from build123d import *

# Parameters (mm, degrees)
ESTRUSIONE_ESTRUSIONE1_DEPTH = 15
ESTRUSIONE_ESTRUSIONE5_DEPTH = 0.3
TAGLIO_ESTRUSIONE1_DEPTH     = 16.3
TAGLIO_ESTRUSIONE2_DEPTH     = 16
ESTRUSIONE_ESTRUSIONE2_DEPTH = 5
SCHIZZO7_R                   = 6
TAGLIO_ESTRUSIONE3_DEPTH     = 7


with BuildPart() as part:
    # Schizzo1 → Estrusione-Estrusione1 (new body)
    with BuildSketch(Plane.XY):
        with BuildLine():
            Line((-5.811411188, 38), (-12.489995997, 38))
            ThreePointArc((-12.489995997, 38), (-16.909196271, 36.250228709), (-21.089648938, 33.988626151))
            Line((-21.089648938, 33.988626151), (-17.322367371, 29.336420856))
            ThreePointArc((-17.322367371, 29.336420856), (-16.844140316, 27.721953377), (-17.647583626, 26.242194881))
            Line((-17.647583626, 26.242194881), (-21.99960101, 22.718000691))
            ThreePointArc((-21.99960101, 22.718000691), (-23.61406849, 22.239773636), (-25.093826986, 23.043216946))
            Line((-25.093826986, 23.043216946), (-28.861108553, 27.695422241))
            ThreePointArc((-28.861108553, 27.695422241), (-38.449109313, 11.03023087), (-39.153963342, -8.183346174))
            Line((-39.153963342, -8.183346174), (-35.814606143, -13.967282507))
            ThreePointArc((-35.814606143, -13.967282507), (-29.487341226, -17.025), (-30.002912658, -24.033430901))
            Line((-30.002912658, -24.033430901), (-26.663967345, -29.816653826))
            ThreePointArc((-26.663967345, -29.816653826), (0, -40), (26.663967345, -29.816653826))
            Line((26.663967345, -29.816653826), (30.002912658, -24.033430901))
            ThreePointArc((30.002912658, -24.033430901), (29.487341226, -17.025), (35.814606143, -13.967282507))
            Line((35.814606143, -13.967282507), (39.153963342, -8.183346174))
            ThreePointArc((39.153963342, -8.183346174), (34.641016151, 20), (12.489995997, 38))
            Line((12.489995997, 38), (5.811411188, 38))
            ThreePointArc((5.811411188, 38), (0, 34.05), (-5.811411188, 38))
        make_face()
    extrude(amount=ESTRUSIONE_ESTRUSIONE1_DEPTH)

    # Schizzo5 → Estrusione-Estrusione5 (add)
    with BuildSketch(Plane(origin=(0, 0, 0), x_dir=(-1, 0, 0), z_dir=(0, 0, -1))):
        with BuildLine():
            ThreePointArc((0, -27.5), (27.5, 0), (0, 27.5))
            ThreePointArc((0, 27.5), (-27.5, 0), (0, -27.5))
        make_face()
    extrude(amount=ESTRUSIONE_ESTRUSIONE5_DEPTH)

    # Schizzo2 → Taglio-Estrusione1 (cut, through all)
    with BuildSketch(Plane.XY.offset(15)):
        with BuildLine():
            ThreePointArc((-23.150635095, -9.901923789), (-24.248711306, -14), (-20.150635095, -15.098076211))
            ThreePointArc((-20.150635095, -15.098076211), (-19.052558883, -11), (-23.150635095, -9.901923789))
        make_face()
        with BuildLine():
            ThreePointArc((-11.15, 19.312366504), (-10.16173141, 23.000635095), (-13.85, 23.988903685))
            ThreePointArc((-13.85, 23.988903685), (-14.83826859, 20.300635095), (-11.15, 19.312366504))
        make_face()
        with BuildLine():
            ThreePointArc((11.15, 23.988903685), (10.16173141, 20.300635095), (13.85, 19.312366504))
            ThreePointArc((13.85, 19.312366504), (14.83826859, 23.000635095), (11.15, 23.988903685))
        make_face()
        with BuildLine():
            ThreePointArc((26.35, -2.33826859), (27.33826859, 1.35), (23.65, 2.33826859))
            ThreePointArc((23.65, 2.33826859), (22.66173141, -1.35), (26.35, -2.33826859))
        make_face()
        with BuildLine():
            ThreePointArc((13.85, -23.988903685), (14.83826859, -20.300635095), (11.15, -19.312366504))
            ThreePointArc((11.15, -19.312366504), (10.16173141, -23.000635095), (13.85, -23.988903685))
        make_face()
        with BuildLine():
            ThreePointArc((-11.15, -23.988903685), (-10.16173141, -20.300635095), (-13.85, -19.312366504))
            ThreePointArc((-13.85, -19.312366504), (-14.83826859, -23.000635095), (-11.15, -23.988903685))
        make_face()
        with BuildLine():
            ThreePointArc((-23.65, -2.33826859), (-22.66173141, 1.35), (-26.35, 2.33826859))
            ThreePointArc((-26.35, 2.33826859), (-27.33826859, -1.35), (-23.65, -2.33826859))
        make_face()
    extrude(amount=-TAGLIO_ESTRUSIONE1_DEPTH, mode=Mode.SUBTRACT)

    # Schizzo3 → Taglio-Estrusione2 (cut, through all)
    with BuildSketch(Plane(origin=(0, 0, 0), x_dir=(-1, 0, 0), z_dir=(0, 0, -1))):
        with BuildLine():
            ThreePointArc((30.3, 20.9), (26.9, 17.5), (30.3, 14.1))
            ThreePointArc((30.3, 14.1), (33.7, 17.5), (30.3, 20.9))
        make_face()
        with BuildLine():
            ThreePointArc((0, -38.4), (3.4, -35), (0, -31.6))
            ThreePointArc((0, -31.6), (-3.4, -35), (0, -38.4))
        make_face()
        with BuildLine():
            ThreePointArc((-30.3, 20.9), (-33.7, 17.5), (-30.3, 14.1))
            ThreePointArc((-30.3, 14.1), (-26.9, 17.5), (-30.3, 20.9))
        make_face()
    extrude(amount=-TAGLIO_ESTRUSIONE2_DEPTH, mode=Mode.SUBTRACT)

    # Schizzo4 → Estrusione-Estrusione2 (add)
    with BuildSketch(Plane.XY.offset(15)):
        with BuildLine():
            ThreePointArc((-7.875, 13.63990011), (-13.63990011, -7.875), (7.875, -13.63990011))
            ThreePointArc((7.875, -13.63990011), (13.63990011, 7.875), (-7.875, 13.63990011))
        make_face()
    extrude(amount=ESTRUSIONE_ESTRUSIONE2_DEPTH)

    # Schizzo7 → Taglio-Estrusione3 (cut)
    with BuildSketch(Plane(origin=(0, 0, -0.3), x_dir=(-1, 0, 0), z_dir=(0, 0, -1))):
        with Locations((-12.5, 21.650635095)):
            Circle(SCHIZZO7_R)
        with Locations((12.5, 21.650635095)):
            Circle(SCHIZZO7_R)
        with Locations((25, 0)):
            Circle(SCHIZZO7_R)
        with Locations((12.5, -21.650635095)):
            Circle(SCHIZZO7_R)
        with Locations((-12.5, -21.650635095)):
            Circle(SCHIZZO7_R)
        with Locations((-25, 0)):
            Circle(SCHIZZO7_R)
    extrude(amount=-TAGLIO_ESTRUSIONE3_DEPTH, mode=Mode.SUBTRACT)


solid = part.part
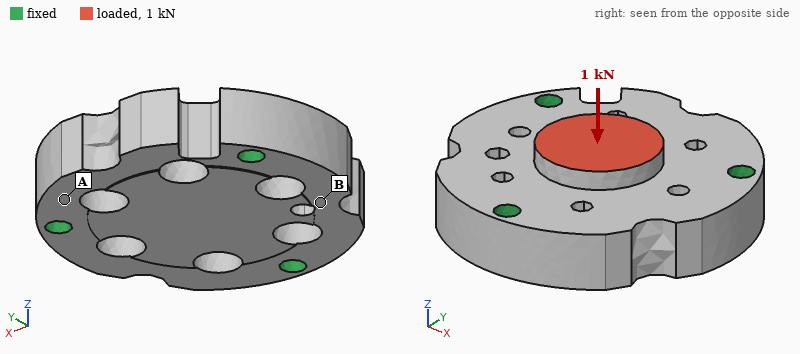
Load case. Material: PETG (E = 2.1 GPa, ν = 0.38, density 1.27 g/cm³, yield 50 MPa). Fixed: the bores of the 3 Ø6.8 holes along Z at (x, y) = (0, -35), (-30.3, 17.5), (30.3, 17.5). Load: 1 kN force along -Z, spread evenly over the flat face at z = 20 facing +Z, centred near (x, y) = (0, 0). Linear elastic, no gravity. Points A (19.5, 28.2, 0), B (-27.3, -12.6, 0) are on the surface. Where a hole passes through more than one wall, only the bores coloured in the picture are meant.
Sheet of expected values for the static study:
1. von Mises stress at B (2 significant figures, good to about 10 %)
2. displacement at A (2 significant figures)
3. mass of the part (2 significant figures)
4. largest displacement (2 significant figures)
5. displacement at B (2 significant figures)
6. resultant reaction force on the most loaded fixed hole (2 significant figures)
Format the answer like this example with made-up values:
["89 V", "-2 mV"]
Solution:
["1.7 MPa", "19 µm", "86 g", "61 µm", "33 µm", "340 N"]
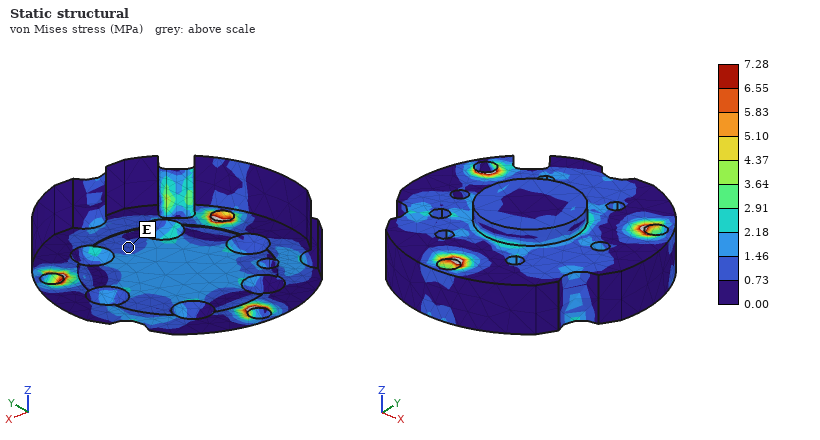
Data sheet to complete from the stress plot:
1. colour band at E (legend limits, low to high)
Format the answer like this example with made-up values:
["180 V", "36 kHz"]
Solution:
["0.73 to 1.46 MPa"]
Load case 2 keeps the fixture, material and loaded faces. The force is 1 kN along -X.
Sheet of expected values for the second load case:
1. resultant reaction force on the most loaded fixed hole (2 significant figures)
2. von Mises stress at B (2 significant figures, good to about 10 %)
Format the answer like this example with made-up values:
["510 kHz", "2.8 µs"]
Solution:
["450 N", "1.3 MPa"]
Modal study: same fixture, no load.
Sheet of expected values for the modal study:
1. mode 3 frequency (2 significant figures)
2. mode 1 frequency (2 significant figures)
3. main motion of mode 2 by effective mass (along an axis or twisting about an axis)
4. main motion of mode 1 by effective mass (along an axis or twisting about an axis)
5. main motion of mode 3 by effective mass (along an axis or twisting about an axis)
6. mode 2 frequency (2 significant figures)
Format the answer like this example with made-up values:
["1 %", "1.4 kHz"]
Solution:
["3400 Hz", "2900 Hz", "along Z", "along Z", "twisting about Y", "3200 Hz"]
